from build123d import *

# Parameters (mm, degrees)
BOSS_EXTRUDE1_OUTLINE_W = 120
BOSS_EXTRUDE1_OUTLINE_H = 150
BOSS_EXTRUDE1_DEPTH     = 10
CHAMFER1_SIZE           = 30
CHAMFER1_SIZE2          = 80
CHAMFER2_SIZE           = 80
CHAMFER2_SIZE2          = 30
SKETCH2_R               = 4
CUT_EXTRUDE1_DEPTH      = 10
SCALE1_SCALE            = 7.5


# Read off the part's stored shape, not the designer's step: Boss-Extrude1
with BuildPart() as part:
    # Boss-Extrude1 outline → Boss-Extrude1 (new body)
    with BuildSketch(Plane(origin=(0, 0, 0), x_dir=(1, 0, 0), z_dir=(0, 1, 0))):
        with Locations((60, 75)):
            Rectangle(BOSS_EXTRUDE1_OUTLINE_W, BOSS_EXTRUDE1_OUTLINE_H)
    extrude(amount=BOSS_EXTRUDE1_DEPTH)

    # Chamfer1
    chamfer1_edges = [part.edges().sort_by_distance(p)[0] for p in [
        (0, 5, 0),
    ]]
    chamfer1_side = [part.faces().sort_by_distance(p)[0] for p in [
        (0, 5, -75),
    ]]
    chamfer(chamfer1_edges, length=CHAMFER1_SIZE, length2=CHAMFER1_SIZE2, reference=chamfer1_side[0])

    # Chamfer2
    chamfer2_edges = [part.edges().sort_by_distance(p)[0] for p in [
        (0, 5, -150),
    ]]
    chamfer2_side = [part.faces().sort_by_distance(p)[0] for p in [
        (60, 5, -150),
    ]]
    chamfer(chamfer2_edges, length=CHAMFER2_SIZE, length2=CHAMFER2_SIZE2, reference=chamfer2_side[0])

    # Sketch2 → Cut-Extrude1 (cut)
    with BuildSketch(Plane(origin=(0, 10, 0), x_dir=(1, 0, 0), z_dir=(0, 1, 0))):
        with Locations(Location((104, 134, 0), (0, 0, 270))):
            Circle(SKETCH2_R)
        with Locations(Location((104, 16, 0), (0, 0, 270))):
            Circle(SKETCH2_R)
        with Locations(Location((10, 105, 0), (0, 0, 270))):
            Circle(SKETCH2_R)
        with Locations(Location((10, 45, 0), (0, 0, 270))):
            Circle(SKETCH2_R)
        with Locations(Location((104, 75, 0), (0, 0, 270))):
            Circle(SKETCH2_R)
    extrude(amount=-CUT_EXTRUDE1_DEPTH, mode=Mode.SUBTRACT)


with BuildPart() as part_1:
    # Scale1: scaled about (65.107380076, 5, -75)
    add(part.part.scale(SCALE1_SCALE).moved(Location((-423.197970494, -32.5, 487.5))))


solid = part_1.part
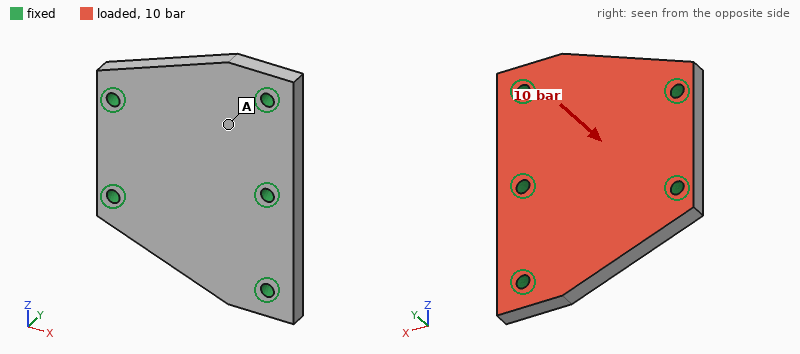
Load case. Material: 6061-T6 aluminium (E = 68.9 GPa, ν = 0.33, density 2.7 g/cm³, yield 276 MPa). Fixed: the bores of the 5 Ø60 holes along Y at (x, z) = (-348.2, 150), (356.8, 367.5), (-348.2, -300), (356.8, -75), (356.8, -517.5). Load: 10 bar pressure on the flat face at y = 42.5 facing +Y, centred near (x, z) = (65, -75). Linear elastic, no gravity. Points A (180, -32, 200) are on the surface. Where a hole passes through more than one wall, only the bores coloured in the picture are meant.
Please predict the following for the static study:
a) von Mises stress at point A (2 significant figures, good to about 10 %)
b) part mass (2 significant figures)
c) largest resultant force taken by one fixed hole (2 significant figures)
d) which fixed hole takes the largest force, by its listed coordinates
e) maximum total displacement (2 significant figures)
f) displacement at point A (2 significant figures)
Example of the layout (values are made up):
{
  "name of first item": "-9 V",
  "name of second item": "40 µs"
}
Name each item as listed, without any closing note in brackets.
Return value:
{
  "von Mises stress at point A": "8.7 MPa",
  "part mass": "170 kg",
  "largest resultant force taken by one fixed hole": "210 kN",
  "which fixed hole takes the largest force, by its listed coordinates": "(356.8, -75)",
  "maximum total displacement": "0.43 mm",
  "displacement at point A": "0.25 mm"
}
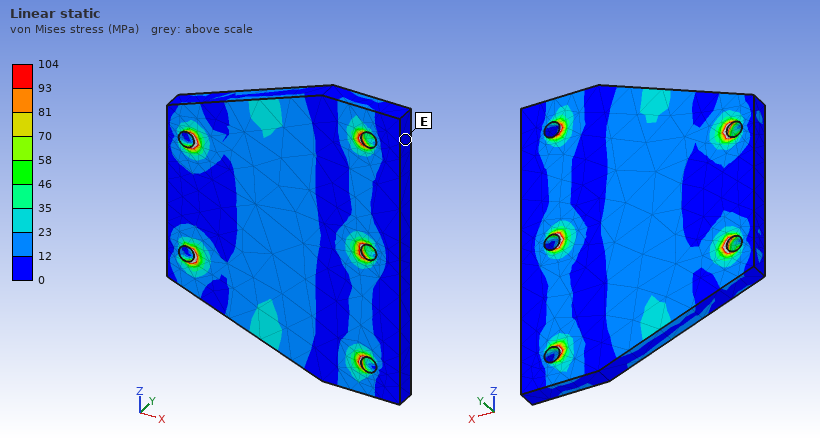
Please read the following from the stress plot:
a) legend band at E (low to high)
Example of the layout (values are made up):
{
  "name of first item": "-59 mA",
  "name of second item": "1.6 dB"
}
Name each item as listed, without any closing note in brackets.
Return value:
{
  "legend band at E": "0 to 12 MPa"
}
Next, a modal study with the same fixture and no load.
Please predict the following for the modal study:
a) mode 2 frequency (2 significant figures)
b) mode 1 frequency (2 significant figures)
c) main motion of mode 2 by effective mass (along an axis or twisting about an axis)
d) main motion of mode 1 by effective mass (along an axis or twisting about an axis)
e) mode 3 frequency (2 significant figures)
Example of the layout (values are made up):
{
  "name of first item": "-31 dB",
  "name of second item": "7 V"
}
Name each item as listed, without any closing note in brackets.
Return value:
{
  "mode 2 frequency": "700 Hz",
  "mode 1 frequency": "640 Hz",
  "main motion of mode 2 by effective mass": "twisting about X",
  "main motion of mode 1 by effective mass": "along Y",
  "mode 3 frequency": "930 Hz"
}
